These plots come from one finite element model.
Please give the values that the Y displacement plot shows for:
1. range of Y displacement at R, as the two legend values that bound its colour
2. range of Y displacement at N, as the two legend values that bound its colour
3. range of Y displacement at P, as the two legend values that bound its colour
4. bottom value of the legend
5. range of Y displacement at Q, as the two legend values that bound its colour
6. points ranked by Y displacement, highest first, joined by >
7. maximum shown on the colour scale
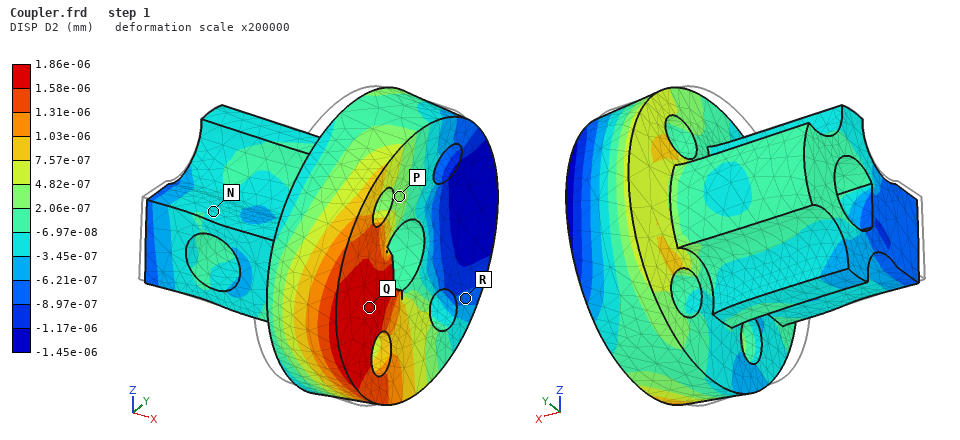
-8.97e-07 to -6.21e-07 mm
-3.45e-07 to -6.97e-08 mm
2.06e-07 to 4.82e-07 mm
-1.45e-06 mm
1.58e-06 to 1.86e-06 mm
Q > P > N > R
1.86e-06 mm
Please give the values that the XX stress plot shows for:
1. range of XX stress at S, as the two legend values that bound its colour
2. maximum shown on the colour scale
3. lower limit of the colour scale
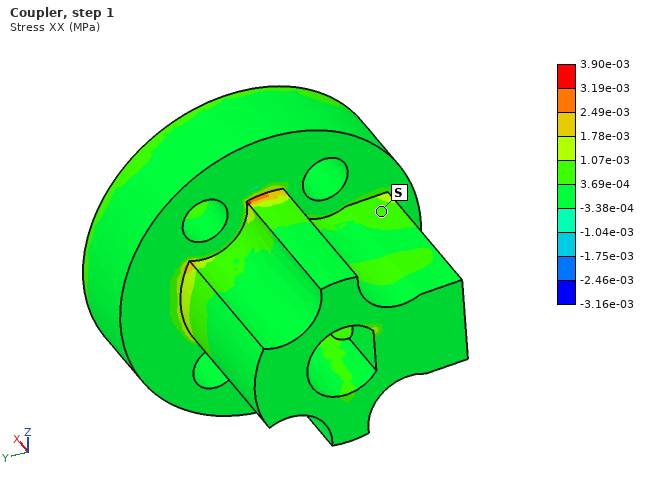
3.69e-04 to 1.07e-03 MPa
3.90e-03 MPa
-3.16e-03 MPa
